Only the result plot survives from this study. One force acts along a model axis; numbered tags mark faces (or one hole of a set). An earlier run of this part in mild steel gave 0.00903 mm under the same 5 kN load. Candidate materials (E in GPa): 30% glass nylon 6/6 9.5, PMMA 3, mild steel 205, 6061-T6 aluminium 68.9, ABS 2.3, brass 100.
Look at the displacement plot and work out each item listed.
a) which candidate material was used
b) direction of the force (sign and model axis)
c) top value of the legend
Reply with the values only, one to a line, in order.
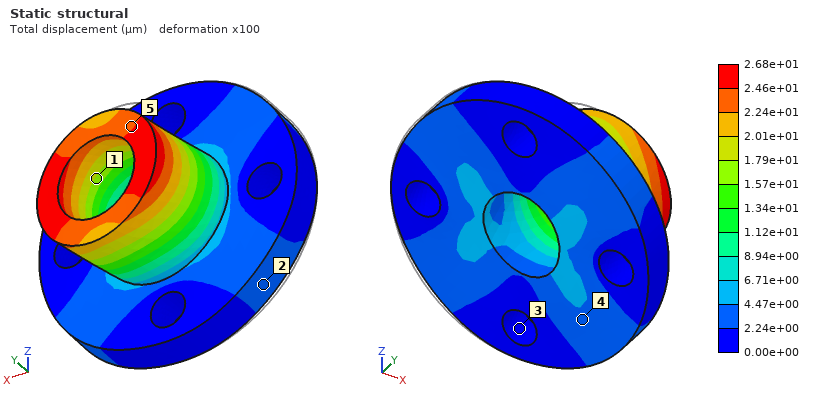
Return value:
6061-T6 aluminium
+X
2.68e+01 µm
